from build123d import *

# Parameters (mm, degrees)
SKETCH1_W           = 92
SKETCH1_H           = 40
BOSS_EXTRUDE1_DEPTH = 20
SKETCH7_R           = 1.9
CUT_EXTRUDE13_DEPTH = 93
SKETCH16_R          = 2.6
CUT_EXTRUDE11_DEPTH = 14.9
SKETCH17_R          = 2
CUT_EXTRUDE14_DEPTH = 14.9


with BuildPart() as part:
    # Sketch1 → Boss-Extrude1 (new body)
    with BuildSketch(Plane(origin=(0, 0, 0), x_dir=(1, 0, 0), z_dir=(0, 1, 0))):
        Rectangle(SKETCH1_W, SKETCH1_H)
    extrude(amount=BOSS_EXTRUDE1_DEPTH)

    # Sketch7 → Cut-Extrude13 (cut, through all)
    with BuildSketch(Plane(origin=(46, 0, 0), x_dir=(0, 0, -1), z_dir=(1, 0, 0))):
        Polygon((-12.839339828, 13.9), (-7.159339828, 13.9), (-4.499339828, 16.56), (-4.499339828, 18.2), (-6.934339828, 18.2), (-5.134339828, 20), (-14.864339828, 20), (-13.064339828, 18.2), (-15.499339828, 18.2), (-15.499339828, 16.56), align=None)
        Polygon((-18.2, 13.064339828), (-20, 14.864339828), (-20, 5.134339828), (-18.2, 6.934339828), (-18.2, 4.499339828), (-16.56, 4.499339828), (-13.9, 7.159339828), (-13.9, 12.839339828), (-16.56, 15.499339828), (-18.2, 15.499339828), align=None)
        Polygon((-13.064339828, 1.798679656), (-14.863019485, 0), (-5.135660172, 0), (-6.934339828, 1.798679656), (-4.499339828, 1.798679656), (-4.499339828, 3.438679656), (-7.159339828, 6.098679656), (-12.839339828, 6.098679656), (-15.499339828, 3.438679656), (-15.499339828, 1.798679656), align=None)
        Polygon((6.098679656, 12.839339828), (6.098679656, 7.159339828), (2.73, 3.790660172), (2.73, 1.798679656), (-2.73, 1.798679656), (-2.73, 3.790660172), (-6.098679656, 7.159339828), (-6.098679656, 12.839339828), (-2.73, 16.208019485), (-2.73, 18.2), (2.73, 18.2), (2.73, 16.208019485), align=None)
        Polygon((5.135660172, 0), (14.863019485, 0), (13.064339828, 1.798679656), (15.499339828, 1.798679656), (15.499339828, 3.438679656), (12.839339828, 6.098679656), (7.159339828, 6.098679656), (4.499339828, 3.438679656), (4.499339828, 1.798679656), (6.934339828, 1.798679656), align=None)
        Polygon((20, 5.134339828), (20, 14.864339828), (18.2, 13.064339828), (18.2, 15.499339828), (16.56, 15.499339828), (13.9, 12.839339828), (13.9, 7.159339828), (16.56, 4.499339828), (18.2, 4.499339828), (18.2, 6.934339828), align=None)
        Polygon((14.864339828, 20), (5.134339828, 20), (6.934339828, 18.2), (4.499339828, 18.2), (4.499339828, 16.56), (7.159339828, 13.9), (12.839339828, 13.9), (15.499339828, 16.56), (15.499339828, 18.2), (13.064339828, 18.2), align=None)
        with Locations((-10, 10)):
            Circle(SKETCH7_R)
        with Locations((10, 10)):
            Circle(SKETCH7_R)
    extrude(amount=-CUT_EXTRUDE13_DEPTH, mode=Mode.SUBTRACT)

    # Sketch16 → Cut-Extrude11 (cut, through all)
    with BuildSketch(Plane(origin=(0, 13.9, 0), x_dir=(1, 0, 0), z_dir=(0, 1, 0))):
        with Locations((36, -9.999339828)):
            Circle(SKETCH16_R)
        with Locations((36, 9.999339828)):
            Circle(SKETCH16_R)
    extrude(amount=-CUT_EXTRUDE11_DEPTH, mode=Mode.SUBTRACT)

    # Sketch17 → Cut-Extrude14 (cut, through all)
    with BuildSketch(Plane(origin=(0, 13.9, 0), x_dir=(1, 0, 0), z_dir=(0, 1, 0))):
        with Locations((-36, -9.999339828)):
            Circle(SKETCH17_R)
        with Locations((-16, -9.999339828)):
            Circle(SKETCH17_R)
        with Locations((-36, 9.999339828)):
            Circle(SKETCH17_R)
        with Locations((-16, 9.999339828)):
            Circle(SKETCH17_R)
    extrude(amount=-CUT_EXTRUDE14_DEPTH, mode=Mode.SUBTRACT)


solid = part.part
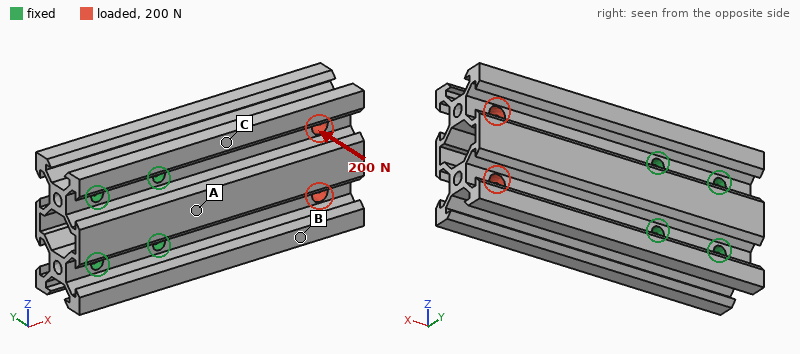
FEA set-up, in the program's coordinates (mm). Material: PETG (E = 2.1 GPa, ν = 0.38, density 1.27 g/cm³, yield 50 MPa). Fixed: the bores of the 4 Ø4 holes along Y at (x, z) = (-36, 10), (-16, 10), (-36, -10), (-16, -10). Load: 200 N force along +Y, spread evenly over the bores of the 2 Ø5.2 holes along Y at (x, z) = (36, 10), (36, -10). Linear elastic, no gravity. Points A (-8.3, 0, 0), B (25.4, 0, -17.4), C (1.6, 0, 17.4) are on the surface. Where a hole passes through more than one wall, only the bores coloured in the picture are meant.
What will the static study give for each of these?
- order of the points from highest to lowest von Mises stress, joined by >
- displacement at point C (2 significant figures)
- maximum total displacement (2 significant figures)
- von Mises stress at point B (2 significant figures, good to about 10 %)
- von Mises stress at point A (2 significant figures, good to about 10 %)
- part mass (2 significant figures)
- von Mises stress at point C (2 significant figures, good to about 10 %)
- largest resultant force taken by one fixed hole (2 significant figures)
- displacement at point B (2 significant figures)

A > C > B
0.23 mm
0.99 mm
1.7 MPa
7.9 MPa
34 g
5.8 MPa
240 N
0.62 mm
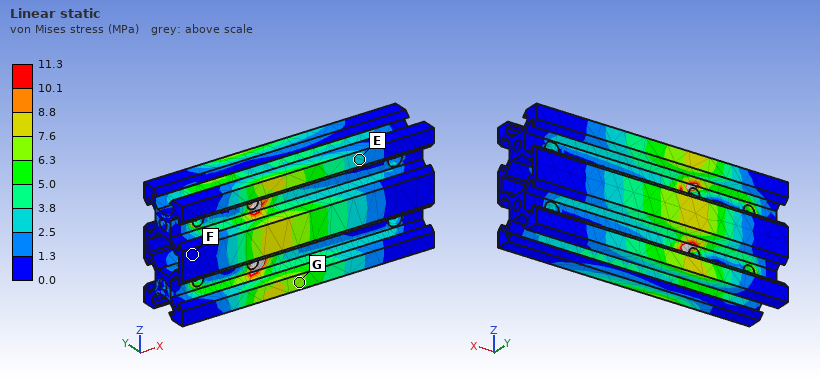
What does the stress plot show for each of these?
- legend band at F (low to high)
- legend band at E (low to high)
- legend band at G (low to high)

0.0 to 1.3 MPa
2.5 to 3.8 MPa
6.3 to 7.6 MPa
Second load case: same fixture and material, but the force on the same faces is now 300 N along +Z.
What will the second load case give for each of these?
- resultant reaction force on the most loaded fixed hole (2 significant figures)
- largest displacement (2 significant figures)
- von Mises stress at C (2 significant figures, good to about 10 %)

460 N
0.54 mm
3.3 MPa
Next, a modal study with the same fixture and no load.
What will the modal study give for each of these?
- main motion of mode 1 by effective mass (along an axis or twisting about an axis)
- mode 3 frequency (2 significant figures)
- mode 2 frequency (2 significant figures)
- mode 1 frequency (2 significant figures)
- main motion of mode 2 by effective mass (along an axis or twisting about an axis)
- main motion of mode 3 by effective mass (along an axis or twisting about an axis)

along Y
1200 Hz
1100 Hz
770 Hz
twisting about X
along Z
